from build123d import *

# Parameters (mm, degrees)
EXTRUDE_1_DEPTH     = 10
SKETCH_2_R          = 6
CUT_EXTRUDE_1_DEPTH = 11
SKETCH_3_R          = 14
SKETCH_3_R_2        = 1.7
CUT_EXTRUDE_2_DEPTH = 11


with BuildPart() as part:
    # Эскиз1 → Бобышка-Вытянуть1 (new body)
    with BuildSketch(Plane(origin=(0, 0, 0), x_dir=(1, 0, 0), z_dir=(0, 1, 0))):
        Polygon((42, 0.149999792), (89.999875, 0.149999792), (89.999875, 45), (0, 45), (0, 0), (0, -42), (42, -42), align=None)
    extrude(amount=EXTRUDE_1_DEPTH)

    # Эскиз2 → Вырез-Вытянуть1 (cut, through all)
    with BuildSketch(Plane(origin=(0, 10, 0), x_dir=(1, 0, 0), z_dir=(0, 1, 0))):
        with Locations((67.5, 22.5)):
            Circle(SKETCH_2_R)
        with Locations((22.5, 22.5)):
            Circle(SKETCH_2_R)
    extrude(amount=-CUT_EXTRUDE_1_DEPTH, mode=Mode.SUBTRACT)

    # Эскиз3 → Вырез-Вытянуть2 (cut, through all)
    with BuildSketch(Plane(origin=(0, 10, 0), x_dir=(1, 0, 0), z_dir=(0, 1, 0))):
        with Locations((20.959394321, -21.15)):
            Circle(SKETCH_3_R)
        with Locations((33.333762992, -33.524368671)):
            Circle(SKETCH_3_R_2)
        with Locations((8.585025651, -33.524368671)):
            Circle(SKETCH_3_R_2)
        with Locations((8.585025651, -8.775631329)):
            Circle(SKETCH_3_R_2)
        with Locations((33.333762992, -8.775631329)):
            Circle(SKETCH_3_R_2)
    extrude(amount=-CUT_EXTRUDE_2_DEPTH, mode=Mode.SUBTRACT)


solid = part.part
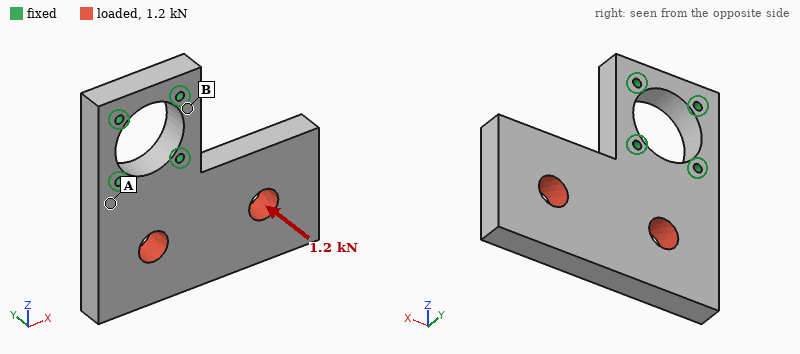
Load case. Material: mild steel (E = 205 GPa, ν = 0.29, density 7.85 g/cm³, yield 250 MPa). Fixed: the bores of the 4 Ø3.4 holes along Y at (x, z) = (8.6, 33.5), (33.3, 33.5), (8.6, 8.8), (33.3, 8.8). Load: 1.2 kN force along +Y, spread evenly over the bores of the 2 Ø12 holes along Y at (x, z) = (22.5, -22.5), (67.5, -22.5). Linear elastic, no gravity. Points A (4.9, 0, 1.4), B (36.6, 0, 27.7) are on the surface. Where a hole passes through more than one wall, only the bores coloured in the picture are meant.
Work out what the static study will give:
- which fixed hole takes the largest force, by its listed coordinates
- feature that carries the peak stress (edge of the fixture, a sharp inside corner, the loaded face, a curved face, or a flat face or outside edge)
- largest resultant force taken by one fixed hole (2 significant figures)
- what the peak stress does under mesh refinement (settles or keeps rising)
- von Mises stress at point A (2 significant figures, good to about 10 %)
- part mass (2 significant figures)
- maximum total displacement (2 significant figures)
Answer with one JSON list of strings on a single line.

["(33.3, 8.8)", "edge of the fixture", "1.6 kN", "keeps rising", "36 MPa", "390 g", "0.11 mm"]
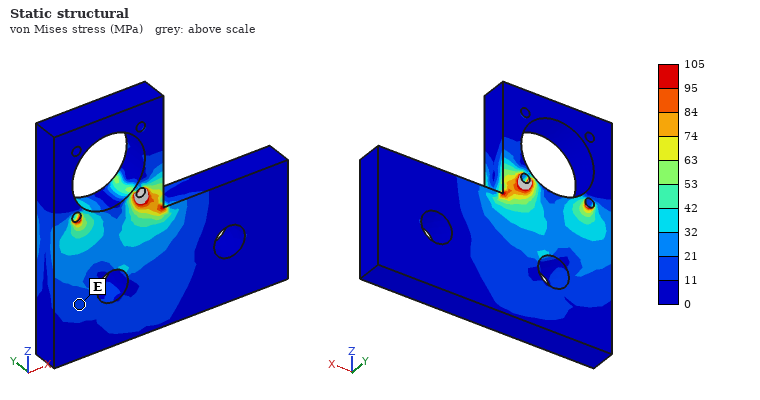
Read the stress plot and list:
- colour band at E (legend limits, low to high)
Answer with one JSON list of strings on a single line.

["11 to 21 MPa"]
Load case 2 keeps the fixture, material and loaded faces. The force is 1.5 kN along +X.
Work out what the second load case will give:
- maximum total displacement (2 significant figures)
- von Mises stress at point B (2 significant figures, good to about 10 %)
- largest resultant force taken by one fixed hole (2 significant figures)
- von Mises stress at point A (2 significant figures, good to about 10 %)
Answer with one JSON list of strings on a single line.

["9.3 µm", "3.4 MPa", "1.6 kN", "8.8 MPa"]
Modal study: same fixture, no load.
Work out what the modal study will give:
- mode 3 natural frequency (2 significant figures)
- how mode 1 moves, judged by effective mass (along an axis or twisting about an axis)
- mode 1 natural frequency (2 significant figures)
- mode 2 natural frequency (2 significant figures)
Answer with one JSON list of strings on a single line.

["3700 Hz", "along Y", "1300 Hz", "2500 Hz"]
